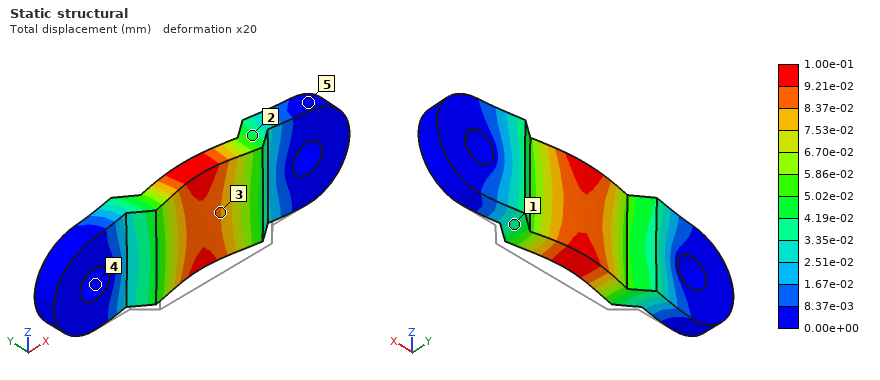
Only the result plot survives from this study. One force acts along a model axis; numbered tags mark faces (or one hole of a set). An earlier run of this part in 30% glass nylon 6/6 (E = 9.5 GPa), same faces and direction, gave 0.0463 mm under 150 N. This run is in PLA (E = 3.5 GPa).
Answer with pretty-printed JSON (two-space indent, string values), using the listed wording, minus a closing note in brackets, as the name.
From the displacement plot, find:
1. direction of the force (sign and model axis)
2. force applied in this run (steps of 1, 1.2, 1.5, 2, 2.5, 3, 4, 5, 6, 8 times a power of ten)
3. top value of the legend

{
  "direction of the force": "+Y",
  "force applied in this run": "120 N",
  "top value of the legend": "1.00e-01 mm"
}
